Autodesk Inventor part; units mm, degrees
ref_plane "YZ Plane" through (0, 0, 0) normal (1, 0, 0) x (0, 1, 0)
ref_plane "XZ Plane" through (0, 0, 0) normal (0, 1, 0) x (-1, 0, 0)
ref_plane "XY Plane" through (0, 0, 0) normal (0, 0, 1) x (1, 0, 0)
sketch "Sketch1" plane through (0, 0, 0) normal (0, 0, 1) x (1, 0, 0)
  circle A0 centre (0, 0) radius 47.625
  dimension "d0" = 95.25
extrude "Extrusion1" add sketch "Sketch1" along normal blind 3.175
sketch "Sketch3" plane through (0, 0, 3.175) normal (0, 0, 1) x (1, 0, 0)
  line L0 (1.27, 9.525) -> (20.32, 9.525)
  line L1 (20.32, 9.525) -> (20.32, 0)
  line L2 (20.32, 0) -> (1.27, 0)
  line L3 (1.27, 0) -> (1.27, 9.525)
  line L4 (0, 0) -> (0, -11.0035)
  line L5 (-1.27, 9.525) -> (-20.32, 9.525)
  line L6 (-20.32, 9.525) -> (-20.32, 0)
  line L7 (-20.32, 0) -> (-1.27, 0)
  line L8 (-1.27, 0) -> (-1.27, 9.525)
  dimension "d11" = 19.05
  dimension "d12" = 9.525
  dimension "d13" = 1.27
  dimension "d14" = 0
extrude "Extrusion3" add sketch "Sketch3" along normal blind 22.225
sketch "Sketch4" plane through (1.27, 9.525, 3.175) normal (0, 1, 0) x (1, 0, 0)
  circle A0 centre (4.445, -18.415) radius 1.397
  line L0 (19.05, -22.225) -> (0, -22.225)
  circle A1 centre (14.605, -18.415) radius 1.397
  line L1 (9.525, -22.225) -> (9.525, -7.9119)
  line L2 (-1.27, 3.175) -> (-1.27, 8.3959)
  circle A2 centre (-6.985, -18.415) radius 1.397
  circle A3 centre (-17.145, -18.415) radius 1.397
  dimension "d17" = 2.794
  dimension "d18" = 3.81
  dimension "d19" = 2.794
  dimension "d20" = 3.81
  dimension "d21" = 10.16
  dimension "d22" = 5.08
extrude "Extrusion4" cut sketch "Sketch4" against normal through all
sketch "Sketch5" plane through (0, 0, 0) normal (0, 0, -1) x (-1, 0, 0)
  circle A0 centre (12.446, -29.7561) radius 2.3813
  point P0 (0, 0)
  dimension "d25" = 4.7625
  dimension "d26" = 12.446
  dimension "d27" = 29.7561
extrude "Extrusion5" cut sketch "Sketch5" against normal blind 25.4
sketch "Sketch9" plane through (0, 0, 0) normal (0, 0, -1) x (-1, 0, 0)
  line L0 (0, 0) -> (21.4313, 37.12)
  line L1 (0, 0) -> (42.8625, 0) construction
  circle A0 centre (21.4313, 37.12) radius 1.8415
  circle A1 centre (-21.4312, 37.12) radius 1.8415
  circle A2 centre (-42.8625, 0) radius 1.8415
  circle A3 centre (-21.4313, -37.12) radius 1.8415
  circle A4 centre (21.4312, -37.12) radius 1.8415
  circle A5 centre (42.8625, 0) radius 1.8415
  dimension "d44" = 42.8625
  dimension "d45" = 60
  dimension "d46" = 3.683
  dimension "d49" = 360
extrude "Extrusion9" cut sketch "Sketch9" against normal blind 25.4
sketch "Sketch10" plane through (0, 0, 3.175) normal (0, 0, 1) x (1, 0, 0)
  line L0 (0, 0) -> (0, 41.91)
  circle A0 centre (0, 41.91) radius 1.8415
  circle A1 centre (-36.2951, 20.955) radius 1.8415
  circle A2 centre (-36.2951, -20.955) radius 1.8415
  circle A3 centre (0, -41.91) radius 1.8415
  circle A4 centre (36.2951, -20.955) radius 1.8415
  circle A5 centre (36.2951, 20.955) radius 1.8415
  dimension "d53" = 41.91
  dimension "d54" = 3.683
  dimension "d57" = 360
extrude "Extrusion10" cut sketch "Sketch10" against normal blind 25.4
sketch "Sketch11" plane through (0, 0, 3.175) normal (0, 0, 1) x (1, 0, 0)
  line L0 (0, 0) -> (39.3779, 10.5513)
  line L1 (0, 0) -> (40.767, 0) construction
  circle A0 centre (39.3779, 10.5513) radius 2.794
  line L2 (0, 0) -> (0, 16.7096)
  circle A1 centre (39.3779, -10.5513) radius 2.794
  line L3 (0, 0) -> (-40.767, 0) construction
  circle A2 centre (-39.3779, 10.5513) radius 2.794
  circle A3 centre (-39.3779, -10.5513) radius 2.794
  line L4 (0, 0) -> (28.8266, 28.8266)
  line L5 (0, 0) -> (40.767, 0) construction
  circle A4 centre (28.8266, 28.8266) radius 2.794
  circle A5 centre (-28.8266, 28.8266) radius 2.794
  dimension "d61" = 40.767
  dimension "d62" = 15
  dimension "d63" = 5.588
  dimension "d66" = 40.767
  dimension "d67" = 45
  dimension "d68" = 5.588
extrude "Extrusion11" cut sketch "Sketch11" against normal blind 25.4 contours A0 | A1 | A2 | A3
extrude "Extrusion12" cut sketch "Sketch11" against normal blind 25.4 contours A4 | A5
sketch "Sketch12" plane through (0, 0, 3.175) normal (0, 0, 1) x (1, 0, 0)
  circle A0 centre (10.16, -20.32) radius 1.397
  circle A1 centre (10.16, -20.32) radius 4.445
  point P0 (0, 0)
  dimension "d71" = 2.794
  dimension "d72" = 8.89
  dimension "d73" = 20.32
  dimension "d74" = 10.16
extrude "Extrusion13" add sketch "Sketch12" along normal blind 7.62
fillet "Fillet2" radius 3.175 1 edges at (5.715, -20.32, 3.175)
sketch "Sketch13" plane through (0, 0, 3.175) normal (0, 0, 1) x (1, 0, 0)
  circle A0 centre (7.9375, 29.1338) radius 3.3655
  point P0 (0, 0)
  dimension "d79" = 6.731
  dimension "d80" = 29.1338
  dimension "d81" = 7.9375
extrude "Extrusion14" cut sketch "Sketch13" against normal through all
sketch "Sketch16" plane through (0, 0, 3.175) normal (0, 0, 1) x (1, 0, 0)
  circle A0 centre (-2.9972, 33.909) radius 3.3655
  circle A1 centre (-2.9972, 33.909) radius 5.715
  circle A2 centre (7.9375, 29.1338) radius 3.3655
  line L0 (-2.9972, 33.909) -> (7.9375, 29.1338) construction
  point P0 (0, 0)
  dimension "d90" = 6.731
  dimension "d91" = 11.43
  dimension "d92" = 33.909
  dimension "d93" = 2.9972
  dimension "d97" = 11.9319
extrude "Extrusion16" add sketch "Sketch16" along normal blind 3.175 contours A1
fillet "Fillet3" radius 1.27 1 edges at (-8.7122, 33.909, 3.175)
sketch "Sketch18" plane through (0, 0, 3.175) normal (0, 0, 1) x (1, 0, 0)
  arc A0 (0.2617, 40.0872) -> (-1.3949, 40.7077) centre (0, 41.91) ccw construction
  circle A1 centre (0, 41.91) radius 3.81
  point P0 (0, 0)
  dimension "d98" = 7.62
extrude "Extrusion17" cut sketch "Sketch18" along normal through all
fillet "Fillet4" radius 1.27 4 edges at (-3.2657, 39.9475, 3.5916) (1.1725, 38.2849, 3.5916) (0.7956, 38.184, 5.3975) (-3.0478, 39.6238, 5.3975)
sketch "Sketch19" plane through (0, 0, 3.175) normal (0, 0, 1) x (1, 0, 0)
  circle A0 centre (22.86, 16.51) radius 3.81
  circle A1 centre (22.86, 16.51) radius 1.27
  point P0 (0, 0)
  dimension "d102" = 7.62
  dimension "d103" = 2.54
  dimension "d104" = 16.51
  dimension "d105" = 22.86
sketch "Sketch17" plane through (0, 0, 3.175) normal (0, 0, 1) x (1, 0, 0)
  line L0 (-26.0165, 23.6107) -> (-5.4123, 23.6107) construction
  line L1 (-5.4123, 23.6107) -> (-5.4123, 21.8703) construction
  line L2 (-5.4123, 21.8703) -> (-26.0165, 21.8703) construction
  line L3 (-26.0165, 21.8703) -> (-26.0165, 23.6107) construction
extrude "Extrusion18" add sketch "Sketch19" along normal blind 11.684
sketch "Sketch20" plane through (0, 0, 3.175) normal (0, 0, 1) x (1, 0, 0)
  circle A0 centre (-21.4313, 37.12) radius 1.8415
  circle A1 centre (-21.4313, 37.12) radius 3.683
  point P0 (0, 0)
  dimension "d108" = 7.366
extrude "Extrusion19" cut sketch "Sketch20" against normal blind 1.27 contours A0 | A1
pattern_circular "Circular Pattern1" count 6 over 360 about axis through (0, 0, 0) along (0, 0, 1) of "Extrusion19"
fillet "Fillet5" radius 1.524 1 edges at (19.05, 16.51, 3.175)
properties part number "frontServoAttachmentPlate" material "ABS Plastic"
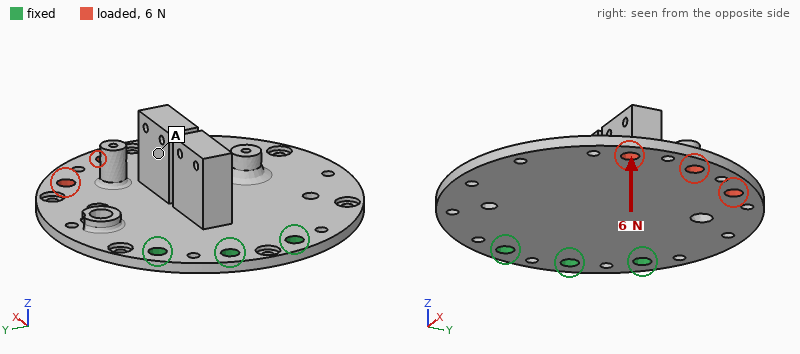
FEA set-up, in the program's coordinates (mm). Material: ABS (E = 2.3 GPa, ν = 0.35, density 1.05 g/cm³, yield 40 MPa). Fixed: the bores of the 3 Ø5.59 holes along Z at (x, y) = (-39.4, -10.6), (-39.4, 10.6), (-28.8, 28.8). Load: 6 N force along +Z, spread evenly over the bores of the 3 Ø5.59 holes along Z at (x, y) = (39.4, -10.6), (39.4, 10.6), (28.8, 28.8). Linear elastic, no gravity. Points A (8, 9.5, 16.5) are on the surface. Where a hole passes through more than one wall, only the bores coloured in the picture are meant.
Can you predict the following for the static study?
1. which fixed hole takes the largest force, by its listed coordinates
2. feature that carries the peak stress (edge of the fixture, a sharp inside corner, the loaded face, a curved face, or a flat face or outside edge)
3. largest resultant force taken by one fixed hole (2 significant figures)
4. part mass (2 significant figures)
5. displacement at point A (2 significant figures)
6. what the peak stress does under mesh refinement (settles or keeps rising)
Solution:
(-28.8, 28.8)
edge of the fixture
8.3 N
32 g
0.61 mm
keeps rising
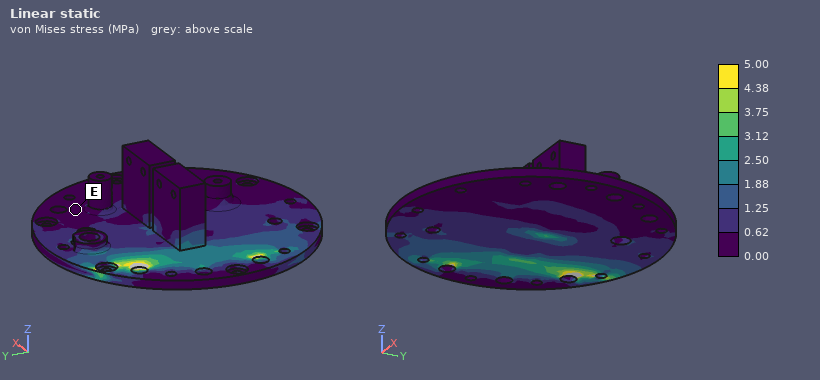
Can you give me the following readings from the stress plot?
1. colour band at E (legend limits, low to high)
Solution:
0.00 to 0.62 MPa
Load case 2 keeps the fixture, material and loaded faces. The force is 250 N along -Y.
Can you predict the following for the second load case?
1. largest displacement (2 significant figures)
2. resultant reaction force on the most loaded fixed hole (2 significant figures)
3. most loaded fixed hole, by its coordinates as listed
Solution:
0.39 mm
430 N
(-28.8, 28.8)
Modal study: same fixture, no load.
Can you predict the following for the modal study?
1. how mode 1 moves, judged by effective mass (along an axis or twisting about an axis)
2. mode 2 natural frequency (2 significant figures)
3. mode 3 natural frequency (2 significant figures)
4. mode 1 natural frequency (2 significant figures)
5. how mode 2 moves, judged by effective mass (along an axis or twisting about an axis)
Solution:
along Z
320 Hz
650 Hz
120 Hz
twisting about X
